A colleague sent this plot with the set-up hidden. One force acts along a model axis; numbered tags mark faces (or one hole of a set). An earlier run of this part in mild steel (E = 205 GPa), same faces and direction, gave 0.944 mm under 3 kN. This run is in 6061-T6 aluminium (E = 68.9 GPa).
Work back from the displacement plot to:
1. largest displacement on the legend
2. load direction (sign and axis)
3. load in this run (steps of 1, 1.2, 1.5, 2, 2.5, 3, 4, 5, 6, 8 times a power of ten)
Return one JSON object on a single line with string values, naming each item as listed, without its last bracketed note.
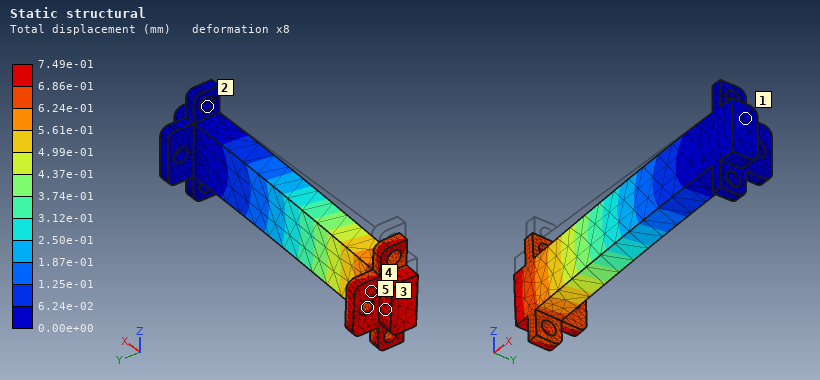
{"largest displacement on the legend": "7.49e-01 mm", "load direction": "-Z", "load in this run": "800 N"}
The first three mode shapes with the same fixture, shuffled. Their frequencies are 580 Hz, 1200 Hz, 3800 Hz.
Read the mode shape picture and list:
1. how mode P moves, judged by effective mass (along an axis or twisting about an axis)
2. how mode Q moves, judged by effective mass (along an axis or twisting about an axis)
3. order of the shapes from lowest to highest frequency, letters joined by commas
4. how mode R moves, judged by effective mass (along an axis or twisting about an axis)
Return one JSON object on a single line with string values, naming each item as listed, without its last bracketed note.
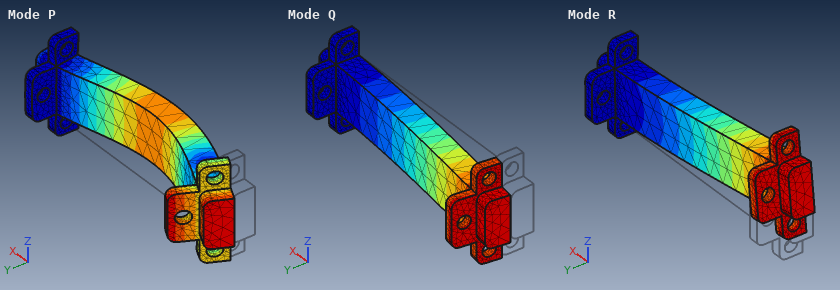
{"how mode P moves, judged by effective mass": "along Y", "how mode Q moves, judged by effective mass": "along Y", "order of the shapes from lowest to highest frequency, letters joined by commas": "Q, R, P", "how mode R moves, judged by effective mass": "along Z"}
